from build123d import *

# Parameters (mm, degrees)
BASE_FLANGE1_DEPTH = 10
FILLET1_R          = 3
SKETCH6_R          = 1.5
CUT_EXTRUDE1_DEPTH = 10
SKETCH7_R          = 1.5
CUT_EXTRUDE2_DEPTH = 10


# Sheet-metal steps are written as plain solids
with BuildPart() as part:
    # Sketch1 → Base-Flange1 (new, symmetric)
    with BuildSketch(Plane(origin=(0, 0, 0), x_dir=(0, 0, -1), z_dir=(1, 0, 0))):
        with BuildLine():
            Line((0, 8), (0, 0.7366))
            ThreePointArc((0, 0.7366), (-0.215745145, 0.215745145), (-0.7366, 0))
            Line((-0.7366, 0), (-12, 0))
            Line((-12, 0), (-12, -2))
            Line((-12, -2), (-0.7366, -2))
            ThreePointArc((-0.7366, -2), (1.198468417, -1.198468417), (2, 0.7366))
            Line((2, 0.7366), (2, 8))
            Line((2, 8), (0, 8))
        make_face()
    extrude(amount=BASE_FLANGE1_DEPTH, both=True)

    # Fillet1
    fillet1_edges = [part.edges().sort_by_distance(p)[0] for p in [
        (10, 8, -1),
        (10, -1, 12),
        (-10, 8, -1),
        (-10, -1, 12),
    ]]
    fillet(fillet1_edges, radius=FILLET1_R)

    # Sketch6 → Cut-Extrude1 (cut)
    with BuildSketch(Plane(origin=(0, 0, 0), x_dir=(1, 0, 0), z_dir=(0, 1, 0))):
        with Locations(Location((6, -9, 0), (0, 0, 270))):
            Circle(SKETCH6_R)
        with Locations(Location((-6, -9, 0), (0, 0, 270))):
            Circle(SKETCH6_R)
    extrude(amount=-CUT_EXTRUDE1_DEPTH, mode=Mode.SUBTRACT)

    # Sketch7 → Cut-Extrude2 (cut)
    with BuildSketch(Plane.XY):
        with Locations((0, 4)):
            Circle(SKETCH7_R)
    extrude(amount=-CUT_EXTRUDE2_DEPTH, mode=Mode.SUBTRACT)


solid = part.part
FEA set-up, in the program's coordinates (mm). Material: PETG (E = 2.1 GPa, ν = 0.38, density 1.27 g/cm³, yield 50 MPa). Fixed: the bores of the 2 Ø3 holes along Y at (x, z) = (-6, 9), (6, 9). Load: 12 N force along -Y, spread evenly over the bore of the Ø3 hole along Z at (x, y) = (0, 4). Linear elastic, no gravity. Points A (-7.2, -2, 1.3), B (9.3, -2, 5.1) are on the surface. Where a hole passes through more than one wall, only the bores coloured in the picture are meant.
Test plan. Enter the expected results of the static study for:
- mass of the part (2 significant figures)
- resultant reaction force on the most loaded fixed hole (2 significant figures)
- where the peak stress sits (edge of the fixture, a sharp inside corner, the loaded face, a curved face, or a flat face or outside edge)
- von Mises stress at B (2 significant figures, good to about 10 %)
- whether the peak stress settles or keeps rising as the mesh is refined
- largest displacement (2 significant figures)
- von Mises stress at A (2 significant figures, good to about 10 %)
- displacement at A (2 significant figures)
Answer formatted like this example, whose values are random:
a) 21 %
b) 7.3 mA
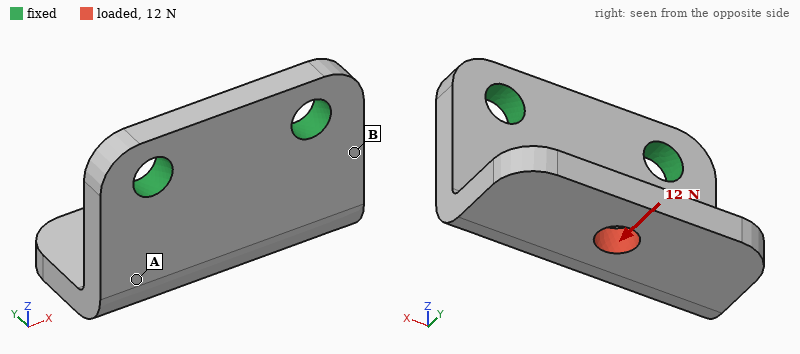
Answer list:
a) 1.0 g
b) 6.0 N
c) edge of the fixture
d) 5.6 MPa
e) keeps rising
f) 0.21 mm
g) 1.9 MPa
h) 0.075 mm
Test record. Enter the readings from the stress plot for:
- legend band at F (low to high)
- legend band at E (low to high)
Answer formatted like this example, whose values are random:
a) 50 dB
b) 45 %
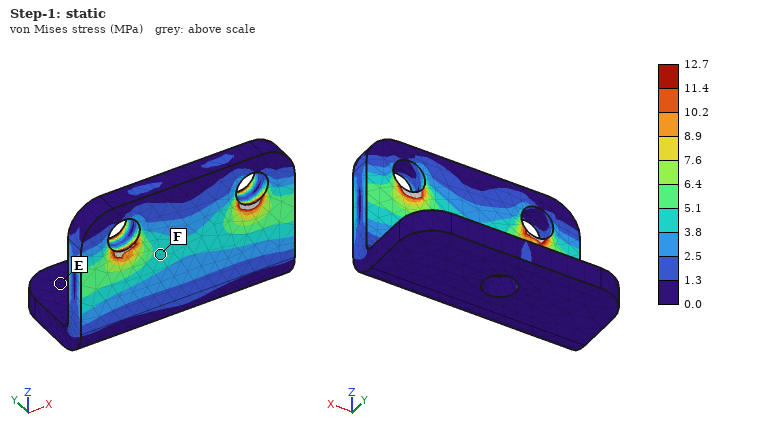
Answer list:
a) 3.8 to 5.1 MPa
b) 0.0 to 1.3 MPa
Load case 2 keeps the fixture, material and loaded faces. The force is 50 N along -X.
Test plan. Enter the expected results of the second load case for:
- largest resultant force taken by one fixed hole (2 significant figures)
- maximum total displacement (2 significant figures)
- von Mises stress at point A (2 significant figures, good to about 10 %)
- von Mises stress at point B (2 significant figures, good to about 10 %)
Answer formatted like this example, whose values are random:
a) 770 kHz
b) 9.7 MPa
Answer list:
a) 46 N
b) 0.31 mm
c) 5.6 MPa
d) 9.3 MPa
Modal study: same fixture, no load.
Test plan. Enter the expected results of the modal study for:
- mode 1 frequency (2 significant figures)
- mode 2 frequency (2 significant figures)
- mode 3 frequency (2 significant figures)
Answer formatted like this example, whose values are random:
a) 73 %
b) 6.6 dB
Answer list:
a) 1800 Hz
b) 2900 Hz
c) 5000 Hz
